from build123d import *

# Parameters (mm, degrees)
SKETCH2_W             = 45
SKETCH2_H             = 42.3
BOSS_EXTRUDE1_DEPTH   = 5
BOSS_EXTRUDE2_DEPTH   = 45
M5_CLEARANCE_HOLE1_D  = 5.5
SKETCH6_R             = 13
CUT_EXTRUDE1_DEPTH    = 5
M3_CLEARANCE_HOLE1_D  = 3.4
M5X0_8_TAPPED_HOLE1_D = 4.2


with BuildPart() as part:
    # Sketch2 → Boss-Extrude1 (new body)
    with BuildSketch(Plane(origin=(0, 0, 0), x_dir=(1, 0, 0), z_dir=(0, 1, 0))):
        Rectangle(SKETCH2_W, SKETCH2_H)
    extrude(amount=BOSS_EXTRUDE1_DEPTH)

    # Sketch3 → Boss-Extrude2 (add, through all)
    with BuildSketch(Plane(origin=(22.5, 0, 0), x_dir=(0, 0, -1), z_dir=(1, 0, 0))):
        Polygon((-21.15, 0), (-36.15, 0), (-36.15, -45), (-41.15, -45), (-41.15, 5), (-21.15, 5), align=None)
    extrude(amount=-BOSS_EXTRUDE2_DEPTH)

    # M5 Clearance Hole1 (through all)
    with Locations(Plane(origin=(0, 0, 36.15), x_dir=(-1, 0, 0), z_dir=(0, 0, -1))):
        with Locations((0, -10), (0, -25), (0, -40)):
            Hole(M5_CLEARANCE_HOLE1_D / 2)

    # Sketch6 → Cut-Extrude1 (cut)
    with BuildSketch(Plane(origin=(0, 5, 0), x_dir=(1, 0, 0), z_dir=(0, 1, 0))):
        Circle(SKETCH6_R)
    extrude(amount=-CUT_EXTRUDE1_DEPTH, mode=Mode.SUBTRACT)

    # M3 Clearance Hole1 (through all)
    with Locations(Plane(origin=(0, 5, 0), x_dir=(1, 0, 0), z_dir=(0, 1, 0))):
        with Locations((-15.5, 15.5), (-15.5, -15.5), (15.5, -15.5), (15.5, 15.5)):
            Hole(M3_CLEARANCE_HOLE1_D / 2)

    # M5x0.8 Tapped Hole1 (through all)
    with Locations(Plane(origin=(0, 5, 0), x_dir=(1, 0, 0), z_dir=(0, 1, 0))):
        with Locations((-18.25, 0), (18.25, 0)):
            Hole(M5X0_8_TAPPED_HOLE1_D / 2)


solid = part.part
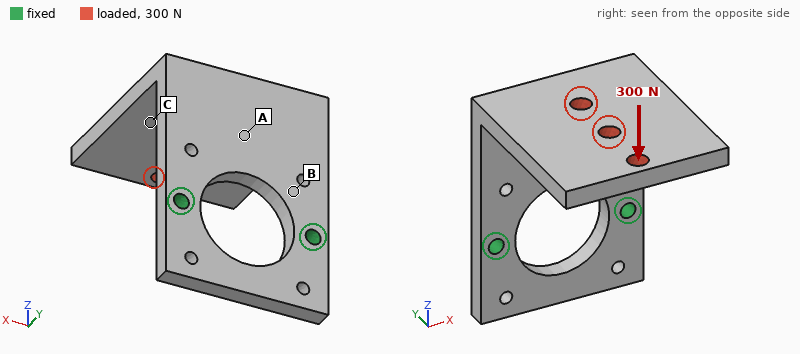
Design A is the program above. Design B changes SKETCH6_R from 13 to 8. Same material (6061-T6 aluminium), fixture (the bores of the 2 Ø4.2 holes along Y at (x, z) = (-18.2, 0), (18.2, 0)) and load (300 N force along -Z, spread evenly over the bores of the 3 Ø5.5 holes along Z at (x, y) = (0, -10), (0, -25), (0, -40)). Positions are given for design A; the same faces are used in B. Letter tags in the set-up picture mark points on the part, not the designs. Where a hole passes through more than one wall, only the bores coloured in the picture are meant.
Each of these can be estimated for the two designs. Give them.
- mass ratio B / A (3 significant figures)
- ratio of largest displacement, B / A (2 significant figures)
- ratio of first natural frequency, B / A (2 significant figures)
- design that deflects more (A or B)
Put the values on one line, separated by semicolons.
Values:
1.08; 0.84; 1.1; A
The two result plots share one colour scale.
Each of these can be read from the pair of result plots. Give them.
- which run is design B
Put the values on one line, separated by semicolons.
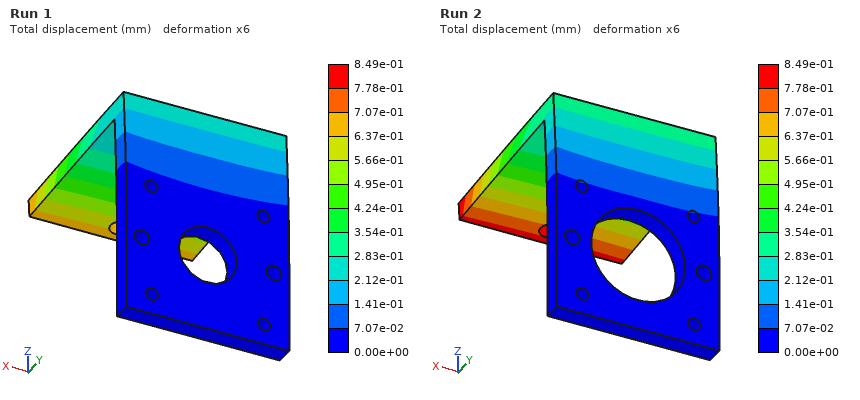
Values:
Run 1
